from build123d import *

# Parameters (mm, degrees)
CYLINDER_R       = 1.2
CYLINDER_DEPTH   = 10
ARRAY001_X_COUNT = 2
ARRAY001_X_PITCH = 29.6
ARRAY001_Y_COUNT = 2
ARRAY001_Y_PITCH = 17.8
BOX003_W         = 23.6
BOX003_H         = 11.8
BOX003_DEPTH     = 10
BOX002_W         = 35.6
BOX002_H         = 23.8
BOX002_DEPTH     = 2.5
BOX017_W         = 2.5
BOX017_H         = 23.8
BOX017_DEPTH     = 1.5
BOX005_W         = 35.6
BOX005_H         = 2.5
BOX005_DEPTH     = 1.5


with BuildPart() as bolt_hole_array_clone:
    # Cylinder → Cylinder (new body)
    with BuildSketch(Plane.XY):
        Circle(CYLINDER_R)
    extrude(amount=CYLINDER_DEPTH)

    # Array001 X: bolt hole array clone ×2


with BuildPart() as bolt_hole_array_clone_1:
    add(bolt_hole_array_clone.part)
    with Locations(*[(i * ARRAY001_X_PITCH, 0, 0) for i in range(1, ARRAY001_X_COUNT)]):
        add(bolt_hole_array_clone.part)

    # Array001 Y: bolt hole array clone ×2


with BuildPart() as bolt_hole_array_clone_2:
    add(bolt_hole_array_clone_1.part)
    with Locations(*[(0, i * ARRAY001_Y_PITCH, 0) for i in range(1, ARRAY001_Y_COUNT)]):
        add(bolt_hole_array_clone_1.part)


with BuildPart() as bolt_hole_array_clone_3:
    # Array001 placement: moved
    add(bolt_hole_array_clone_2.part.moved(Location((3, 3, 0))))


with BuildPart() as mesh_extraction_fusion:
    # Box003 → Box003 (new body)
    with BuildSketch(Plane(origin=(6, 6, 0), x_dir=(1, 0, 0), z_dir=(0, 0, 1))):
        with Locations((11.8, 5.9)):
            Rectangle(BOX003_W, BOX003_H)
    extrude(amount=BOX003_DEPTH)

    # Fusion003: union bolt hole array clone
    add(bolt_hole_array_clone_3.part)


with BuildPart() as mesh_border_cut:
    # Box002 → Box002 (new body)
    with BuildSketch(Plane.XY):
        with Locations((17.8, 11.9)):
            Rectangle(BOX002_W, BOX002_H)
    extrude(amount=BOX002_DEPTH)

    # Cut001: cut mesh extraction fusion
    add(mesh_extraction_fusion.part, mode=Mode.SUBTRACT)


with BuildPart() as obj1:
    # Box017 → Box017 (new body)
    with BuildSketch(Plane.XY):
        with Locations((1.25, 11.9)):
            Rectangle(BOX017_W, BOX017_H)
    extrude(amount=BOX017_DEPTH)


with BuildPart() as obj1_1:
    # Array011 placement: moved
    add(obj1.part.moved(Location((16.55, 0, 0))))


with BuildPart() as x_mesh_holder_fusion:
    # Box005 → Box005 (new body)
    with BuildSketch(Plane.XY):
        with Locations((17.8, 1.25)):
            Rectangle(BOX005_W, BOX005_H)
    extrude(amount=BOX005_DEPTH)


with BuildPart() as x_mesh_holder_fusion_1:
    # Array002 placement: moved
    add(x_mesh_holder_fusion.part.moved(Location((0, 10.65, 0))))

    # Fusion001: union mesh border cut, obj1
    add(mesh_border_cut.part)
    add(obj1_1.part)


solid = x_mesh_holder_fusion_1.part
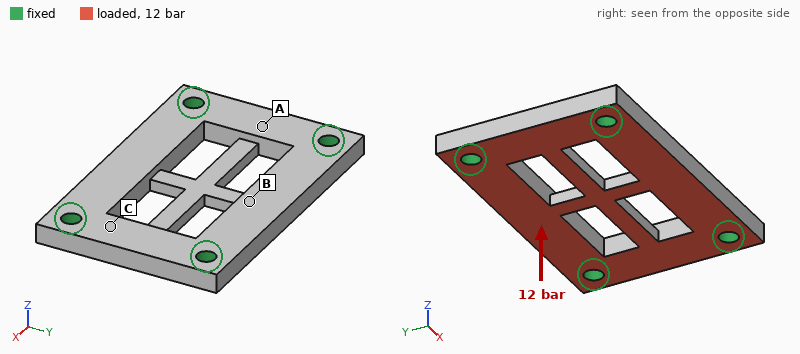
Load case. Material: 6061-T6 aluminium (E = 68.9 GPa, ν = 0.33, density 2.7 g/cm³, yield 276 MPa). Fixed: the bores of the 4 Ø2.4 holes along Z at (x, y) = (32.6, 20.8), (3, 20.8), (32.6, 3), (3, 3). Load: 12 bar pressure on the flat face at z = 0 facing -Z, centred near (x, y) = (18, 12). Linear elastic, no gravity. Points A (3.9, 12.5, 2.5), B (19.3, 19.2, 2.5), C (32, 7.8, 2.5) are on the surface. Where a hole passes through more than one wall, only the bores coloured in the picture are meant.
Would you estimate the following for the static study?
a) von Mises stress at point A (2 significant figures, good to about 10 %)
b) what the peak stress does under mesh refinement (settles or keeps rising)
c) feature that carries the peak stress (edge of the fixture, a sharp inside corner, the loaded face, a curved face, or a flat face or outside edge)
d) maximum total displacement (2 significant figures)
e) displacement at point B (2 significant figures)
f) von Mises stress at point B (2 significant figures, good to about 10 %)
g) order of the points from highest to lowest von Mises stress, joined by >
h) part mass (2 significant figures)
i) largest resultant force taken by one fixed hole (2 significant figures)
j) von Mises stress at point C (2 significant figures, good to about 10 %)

27 MPa
keeps rising
edge of the fixture
45 µm
31 µm
51 MPa
B > A > C
4.1 g
190 N
14 MPa
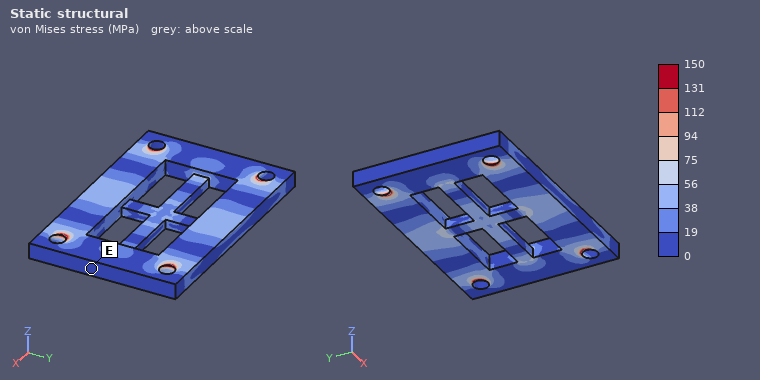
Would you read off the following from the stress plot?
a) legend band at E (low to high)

0 to 19 MPa
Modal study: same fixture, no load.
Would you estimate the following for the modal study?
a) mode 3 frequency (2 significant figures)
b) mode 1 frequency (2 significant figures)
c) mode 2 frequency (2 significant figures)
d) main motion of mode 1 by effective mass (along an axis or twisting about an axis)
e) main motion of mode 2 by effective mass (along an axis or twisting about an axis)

23 kHz
14 kHz
16 kHz
along Z
twisting about X
